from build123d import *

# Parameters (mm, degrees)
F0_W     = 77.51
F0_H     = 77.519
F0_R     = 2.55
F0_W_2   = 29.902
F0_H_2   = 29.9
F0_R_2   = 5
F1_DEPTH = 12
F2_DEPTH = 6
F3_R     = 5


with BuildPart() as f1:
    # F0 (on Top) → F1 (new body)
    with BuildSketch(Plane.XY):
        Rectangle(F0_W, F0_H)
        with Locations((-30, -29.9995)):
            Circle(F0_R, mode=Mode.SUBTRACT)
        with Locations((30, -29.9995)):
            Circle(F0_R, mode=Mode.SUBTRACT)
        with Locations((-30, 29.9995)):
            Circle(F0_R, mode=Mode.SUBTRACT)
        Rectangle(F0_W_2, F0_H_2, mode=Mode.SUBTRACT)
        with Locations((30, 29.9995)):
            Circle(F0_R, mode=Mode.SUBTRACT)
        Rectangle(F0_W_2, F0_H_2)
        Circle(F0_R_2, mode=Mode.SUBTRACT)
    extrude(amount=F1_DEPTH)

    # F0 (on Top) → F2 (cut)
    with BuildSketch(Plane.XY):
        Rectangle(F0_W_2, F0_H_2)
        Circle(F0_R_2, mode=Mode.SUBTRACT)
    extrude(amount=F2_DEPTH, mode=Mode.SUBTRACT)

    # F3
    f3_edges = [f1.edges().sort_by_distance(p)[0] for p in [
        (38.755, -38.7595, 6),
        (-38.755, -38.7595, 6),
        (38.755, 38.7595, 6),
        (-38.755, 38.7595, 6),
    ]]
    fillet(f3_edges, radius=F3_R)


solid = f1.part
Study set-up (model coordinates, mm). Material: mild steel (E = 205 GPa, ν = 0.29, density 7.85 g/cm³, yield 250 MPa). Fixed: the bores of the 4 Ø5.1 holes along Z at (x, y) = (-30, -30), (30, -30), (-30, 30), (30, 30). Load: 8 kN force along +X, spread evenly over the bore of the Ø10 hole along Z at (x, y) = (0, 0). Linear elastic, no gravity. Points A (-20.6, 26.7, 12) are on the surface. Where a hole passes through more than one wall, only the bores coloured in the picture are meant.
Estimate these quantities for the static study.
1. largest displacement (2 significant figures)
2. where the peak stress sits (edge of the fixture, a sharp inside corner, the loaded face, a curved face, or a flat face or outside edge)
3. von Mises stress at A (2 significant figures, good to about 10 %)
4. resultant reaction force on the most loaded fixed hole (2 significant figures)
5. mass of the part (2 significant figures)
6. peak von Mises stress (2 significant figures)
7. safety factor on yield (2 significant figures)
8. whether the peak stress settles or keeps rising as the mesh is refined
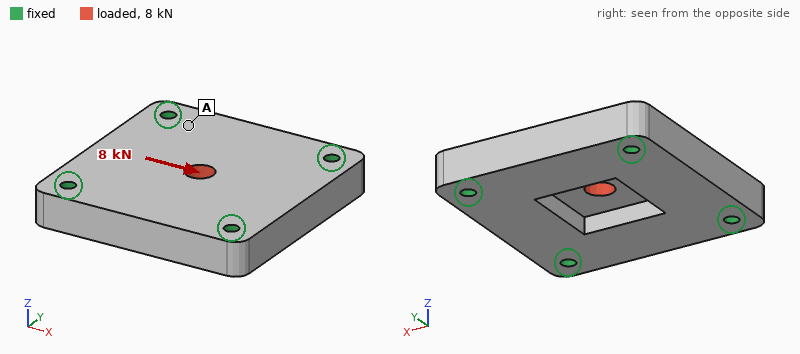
4.1 µm
the loaded face
12 MPa
2.2 kN
510 g
75 MPa
3.3
settles
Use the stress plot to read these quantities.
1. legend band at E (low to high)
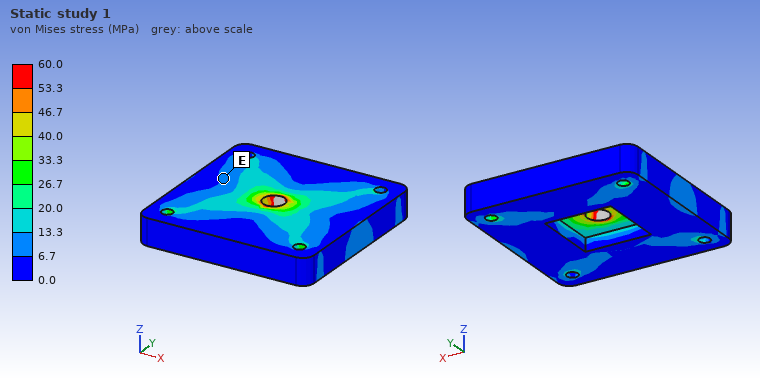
6.7 to 13.3 MPa
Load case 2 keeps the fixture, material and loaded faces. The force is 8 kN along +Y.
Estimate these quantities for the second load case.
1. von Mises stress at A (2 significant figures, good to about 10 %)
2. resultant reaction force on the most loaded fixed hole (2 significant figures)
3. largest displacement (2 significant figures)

12 MPa
2.2 kN
4.1 µm
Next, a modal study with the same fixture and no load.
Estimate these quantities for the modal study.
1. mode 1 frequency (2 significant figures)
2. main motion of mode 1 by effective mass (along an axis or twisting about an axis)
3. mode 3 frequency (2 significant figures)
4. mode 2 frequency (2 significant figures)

9900 Hz
along Z
15 kHz
15 kHz
